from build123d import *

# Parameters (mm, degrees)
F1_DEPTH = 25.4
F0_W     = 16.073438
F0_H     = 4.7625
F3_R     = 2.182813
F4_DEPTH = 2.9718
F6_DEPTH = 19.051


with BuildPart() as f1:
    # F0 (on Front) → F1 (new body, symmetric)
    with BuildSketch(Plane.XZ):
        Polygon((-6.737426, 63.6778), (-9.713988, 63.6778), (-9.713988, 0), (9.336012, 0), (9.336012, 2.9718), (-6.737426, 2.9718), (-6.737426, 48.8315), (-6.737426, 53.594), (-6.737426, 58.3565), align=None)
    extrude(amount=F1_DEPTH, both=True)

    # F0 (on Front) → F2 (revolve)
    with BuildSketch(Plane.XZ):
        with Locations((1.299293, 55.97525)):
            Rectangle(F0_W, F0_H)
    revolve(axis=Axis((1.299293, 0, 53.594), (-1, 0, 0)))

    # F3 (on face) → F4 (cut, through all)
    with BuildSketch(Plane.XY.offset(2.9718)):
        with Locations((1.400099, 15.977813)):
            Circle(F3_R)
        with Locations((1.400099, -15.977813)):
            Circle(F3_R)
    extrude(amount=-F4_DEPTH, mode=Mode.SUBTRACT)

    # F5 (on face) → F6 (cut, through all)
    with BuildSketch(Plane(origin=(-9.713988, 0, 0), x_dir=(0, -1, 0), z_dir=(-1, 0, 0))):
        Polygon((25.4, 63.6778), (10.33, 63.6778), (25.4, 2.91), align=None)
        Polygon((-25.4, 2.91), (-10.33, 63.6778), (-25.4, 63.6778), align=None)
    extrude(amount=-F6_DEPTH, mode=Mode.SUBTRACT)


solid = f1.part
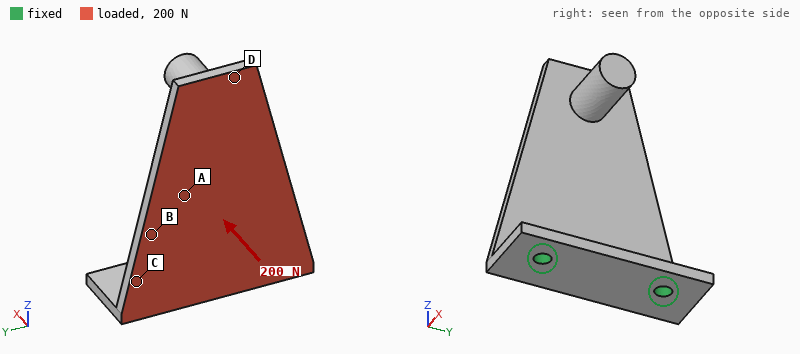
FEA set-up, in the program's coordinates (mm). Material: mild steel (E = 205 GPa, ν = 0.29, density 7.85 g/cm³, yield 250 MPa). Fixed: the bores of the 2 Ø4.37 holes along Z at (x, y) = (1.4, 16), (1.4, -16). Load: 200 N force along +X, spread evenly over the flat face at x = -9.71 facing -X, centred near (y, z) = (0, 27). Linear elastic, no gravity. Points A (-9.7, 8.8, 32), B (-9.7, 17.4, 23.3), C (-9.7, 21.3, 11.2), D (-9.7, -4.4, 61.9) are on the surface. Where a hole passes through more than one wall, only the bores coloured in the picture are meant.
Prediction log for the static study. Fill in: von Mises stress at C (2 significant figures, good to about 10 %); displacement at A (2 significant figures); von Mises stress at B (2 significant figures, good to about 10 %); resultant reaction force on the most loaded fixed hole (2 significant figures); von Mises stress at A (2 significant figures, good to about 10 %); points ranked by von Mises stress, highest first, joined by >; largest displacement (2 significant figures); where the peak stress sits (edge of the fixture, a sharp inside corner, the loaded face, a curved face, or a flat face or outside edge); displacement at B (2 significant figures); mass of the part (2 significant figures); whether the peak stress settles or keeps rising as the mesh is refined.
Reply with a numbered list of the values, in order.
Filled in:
1. 53 MPa
2. 0.14 mm
3. 35 MPa
4. 100 N
5. 22 MPa
6. C > B > A > D
7. 0.35 mm
8. edge of the fixture
9. 0.085 mm
10. 82 g
11. keeps rising
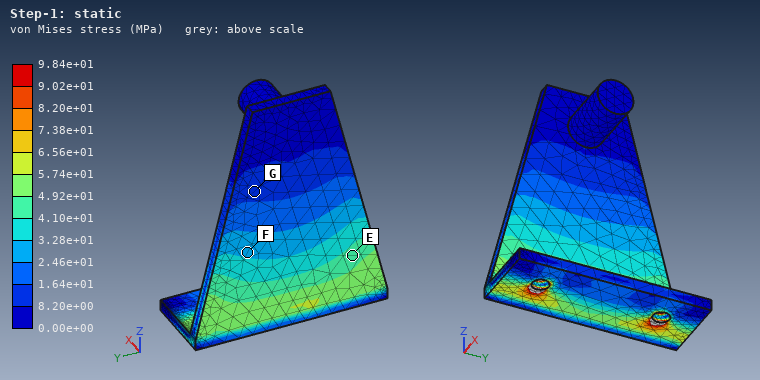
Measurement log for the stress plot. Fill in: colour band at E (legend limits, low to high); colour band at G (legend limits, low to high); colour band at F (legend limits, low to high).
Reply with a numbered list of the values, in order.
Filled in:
1. 4.10e+01 to 4.92e+01 MPa
2. 8.20e+00 to 1.64e+01 MPa
3. 2.46e+01 to 3.28e+01 MPa
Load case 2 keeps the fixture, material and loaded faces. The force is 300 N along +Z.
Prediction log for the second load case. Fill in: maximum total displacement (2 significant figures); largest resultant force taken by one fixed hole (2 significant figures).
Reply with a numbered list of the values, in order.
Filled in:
1. 75 µm
2. 150 N
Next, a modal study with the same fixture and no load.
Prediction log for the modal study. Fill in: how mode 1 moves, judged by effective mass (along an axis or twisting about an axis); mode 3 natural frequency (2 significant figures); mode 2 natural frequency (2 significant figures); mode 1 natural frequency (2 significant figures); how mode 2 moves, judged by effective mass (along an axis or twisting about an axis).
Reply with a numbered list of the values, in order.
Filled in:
1. along X
2. 2800 Hz
3. 2000 Hz
4. 540 Hz
5. along Y
